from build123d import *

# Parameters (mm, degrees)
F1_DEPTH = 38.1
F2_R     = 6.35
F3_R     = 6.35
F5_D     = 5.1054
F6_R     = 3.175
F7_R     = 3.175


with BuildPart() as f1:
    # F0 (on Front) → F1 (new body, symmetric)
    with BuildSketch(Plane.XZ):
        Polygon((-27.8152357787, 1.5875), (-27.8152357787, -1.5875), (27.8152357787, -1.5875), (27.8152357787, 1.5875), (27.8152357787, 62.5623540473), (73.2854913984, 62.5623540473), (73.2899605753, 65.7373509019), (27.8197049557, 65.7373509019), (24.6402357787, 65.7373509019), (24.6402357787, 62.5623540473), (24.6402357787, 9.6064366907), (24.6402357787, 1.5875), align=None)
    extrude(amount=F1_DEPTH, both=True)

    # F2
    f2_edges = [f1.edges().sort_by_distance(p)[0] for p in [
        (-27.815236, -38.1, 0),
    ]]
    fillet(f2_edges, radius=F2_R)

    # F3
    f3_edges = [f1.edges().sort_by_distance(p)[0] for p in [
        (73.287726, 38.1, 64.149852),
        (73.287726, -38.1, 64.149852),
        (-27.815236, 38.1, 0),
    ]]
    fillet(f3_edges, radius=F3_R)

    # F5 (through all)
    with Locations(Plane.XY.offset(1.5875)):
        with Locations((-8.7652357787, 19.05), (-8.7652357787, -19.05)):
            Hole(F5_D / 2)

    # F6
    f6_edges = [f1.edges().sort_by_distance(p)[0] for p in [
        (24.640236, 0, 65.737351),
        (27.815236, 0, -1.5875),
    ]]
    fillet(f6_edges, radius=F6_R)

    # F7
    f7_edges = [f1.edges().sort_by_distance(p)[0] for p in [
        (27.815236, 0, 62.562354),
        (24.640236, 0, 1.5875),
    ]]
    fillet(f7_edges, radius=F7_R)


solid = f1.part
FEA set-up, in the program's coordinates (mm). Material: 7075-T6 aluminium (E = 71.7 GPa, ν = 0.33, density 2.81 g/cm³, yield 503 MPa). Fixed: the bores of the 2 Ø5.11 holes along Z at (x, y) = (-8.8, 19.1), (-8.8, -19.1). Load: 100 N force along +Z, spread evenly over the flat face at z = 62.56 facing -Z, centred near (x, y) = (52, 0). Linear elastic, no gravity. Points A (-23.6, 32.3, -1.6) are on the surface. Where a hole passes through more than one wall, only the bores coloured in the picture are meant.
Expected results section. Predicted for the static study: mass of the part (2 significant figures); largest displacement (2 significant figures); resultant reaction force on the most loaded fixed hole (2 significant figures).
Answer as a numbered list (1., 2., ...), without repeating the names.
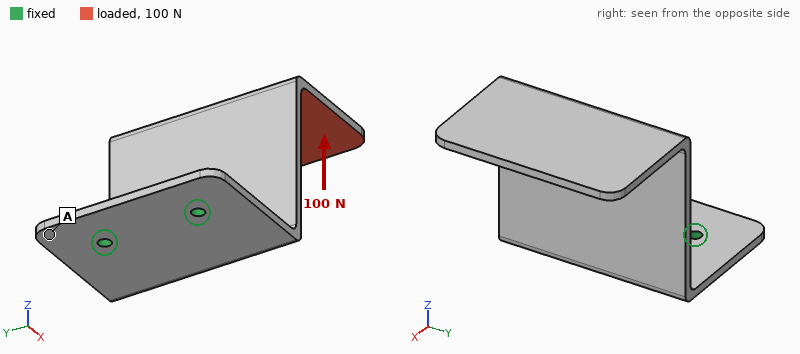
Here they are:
1. 110 g
2. 1.5 mm
3. 51 N
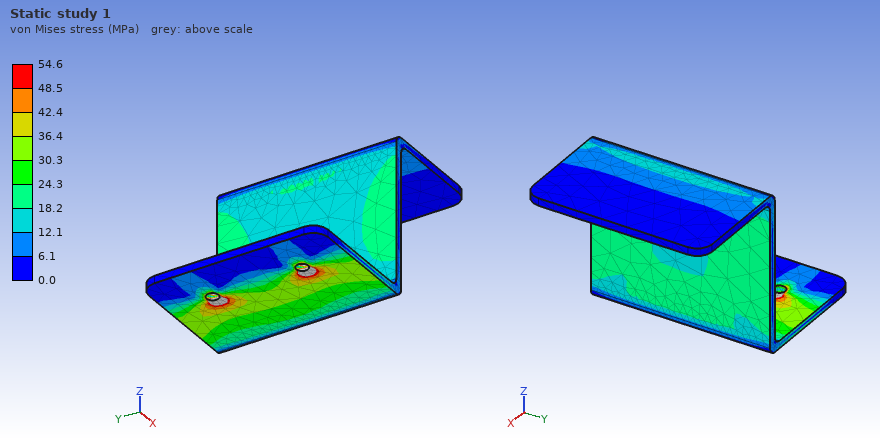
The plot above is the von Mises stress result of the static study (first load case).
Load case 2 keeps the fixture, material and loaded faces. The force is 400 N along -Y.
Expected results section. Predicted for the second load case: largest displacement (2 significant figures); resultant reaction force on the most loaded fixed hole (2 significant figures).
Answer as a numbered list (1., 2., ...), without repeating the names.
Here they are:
1. 1.5 mm
2. 820 N
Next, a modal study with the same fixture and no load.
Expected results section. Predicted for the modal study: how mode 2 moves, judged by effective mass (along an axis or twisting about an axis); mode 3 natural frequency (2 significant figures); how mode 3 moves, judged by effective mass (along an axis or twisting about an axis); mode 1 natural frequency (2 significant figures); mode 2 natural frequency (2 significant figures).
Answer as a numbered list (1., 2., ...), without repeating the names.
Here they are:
1. along Y
2. 590 Hz
3. twisting about Z
4. 170 Hz
5. 430 Hz
